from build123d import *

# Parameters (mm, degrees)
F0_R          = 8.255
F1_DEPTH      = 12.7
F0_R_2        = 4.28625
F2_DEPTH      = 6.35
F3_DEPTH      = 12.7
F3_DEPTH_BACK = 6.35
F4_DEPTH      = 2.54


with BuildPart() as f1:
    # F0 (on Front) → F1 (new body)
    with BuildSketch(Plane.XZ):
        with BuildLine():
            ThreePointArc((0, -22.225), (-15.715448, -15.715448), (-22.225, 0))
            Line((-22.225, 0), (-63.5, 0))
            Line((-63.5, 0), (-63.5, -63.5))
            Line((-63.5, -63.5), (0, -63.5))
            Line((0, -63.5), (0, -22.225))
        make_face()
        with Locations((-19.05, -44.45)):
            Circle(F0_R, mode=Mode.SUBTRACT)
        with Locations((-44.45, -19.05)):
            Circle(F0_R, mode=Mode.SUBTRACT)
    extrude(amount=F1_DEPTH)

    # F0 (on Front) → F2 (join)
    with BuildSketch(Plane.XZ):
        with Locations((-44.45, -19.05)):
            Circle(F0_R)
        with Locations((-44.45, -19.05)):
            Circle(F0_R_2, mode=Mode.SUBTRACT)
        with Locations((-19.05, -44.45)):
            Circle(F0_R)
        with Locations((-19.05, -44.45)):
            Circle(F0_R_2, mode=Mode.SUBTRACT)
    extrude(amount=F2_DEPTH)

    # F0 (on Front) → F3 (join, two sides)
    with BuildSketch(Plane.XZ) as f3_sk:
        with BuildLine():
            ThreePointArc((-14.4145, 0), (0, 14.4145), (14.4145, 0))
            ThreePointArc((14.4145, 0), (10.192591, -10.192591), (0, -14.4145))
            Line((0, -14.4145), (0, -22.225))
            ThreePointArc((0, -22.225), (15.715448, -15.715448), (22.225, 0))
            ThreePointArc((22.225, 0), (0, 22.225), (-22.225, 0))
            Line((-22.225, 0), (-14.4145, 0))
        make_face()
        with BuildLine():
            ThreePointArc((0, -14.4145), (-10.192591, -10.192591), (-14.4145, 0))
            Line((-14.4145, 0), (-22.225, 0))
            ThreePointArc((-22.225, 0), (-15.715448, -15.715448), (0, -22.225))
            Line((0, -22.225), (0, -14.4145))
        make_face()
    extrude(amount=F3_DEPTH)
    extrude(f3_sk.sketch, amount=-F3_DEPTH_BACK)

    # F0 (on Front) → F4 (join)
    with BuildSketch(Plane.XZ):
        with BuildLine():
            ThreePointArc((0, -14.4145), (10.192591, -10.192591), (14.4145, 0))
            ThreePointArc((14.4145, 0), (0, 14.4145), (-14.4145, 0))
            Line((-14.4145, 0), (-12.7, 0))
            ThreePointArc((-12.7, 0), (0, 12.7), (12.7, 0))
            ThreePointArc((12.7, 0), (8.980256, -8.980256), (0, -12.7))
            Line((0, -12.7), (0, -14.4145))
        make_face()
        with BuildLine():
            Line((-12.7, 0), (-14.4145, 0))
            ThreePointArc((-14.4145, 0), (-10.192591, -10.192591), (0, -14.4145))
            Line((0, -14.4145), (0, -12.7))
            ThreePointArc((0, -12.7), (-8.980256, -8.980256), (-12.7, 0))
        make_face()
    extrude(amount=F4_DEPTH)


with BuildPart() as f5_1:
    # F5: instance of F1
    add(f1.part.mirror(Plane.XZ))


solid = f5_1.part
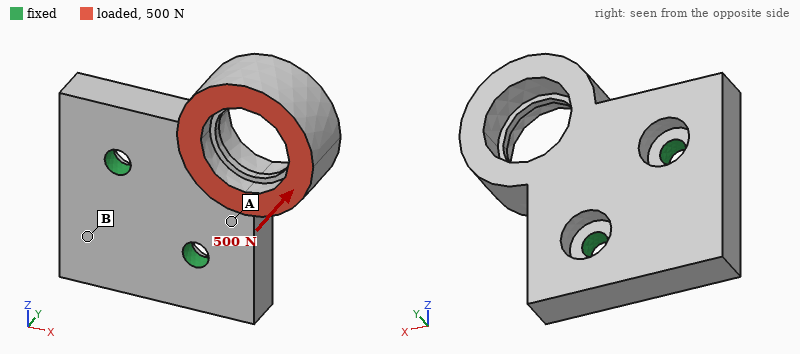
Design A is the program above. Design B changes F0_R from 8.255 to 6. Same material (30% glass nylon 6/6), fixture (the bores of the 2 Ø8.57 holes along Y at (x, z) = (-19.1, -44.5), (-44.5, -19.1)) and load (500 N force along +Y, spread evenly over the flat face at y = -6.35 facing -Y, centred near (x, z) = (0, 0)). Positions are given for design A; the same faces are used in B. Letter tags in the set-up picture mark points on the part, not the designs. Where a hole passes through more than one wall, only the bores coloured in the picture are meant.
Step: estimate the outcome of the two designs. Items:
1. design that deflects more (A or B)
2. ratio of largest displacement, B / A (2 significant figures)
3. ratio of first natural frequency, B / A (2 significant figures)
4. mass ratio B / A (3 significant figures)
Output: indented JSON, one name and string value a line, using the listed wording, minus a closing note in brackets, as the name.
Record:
{
  "design that deflects more": "A",
  "ratio of largest displacement, B / A": "0.92",
  "ratio of first natural frequency, B / A": "1.0",
  "mass ratio B / A": "1.02"
}
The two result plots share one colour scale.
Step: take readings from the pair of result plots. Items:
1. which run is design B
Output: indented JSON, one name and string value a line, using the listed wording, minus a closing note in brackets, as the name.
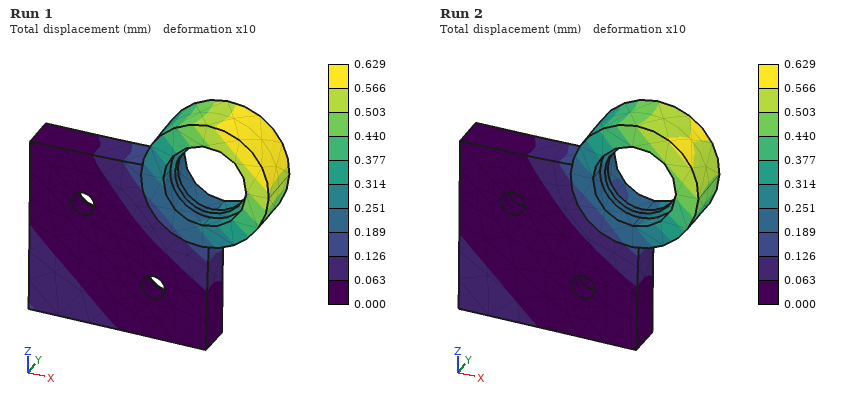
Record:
{
  "which run is design B": "Run 2"
}
